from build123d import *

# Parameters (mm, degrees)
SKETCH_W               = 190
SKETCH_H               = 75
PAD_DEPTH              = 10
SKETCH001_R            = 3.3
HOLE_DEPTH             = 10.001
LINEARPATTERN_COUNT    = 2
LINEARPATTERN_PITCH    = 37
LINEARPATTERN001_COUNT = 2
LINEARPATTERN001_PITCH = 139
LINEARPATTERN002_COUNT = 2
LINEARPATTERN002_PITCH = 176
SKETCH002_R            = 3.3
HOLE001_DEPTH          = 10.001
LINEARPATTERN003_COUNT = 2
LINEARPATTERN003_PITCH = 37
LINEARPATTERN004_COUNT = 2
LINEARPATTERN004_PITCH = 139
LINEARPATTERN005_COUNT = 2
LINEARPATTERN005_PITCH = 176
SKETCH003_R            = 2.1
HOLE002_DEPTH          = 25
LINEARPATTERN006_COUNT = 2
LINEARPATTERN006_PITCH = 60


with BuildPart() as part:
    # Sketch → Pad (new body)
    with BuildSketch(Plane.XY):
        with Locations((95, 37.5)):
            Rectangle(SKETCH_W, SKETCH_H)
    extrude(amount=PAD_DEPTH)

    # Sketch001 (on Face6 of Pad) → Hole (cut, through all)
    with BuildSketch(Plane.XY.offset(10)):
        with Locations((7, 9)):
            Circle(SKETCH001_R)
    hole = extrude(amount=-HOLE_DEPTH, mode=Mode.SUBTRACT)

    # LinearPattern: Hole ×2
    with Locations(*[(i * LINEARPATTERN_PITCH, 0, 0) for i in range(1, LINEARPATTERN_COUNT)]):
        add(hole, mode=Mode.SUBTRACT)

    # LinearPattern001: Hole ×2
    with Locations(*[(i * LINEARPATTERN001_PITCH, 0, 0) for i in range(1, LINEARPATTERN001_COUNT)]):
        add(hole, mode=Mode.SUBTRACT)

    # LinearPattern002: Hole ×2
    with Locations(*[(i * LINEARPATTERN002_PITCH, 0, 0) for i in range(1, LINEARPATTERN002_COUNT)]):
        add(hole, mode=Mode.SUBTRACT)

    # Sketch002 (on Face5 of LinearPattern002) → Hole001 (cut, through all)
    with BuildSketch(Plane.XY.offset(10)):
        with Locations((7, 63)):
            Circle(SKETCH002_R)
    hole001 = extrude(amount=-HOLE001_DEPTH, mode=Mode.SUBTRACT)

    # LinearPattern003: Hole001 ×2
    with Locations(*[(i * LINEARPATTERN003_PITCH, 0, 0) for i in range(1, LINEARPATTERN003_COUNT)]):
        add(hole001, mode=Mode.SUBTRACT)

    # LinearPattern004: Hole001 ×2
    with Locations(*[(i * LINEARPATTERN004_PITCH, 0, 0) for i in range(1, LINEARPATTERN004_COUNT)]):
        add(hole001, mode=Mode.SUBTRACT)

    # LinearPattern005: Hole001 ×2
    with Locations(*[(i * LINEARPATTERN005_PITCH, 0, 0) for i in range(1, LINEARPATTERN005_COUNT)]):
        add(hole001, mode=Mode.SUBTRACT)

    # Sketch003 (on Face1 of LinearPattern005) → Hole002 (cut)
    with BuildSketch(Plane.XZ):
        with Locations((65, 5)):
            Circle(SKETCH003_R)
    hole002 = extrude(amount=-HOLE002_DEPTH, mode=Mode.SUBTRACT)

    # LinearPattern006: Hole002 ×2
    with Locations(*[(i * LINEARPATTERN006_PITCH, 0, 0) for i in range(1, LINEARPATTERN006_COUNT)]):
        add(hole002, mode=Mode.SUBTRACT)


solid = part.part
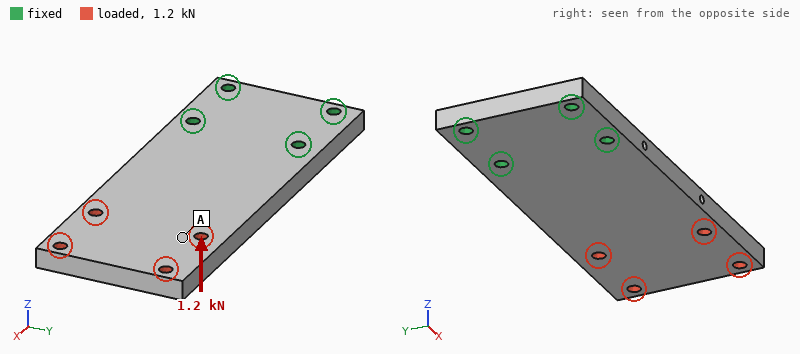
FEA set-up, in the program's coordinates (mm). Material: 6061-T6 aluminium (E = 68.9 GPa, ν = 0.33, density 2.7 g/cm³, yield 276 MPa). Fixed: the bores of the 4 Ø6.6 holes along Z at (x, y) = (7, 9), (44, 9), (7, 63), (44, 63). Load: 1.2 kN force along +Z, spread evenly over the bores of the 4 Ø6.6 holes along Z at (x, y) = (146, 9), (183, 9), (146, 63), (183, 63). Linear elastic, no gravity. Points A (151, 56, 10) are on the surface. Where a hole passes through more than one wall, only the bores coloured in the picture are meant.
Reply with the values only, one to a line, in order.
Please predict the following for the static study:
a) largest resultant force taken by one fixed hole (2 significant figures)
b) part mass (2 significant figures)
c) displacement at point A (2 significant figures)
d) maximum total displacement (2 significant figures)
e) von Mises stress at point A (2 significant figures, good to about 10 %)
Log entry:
1.3 kN
380 g
1.4 mm
2.2 mm
19 MPa
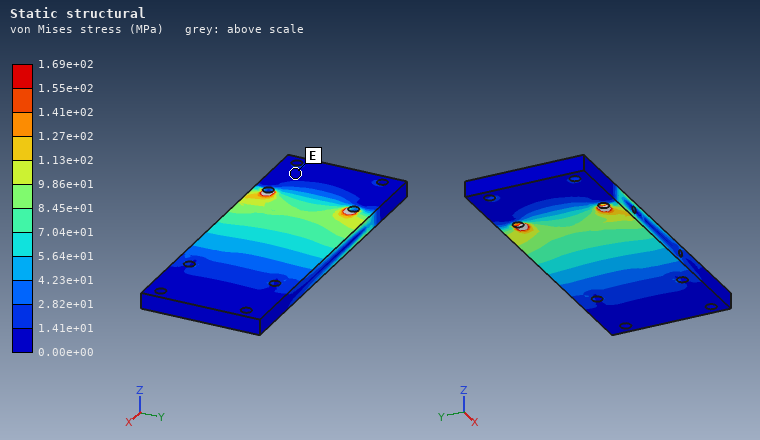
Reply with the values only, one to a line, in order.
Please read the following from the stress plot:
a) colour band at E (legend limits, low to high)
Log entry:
0.00e+00 to 1.41e+01 MPa
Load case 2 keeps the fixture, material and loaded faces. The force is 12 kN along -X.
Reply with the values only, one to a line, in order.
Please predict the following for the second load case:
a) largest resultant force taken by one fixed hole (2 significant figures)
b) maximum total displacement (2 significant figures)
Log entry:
5.1 kN
43 µm
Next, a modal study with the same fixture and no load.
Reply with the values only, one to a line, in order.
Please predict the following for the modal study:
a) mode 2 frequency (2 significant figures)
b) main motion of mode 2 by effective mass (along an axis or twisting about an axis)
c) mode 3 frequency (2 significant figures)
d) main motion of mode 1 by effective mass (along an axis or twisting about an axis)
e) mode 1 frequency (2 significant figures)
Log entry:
1600 Hz
twisting about X
2300 Hz
along Z
380 Hz
